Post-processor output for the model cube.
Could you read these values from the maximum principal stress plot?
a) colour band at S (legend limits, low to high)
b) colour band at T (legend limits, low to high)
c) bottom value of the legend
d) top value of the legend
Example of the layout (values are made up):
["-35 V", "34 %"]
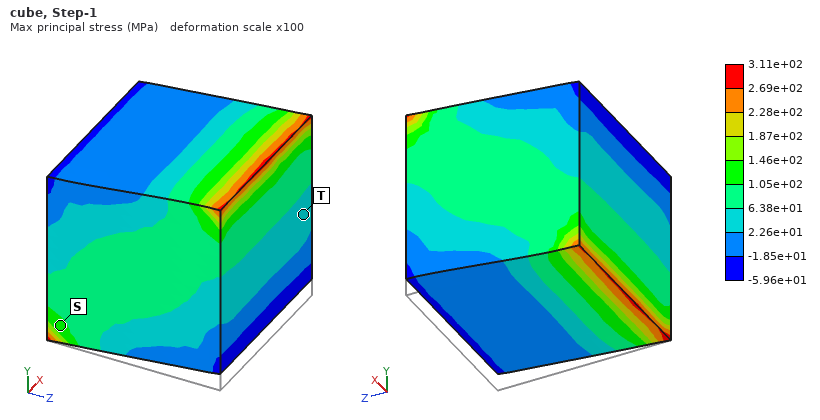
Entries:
["1.05e+02 to 1.46e+02 MPa", "2.26e+01 to 6.38e+01 MPa", "-5.96e+01 MPa", "3.11e+02 MPa"]
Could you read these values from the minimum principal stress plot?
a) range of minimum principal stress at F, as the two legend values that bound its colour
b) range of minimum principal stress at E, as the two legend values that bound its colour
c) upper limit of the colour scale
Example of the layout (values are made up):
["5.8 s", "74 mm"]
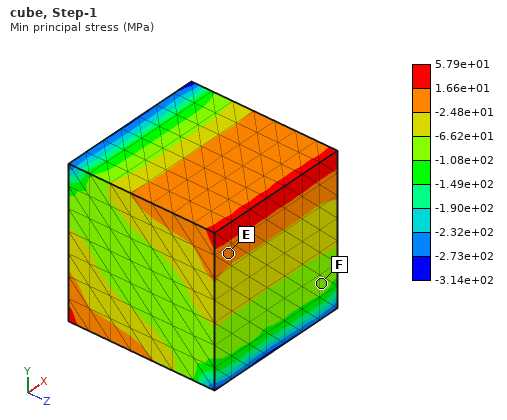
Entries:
["-1.08e+02 to -6.62e+01 MPa", "-2.48e+01 to 1.66e+01 MPa", "5.79e+01 MPa"]
